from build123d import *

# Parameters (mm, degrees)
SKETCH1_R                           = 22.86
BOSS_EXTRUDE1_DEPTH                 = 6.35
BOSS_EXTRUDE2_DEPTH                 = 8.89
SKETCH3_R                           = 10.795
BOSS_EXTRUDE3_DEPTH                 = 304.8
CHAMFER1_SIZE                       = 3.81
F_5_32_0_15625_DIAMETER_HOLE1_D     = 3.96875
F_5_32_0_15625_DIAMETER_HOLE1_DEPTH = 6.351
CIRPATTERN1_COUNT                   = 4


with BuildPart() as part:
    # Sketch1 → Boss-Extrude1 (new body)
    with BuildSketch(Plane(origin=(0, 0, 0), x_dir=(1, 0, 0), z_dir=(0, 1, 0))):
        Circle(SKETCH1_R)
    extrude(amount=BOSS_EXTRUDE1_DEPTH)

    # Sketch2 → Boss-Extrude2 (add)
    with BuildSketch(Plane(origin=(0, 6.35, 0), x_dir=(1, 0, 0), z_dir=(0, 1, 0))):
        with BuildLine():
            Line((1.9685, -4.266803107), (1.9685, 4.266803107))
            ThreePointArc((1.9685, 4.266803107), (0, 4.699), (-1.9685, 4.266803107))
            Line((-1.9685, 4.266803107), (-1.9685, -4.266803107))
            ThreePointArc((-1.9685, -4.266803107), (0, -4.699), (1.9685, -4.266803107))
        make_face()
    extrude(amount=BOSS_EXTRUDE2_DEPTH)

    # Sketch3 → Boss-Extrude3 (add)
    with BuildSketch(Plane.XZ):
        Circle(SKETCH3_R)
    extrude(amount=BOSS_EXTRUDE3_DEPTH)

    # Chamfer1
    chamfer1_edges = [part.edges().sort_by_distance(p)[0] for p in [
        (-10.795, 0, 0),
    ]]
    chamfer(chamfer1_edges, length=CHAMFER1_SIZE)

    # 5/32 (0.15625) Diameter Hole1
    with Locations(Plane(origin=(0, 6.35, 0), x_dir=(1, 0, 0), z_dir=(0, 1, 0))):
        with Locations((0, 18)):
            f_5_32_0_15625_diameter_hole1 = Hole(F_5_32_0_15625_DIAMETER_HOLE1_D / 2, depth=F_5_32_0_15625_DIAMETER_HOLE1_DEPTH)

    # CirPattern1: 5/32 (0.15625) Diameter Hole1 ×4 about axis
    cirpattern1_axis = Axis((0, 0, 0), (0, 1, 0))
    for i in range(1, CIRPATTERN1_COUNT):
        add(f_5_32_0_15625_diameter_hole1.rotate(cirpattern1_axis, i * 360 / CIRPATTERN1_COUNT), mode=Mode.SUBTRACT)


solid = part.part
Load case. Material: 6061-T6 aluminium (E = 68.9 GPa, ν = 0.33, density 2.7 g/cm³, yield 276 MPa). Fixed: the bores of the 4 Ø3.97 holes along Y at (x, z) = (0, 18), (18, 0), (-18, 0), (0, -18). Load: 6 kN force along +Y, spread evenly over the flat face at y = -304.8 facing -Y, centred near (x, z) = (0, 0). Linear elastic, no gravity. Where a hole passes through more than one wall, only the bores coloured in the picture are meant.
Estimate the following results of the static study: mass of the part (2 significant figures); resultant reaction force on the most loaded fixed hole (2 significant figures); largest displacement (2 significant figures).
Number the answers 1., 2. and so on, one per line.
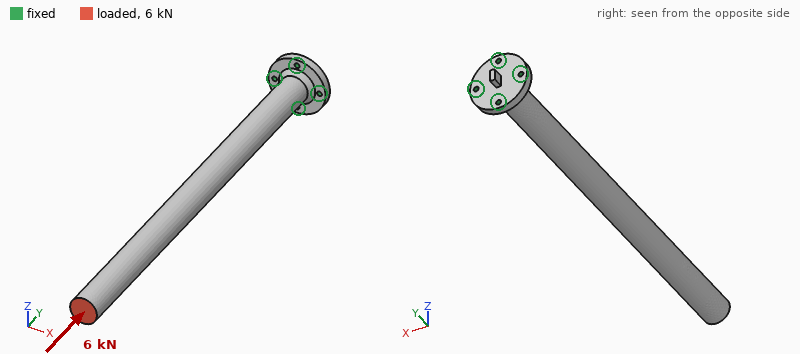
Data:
1. 330 g
2. 1.6 kN
3. 80 µm
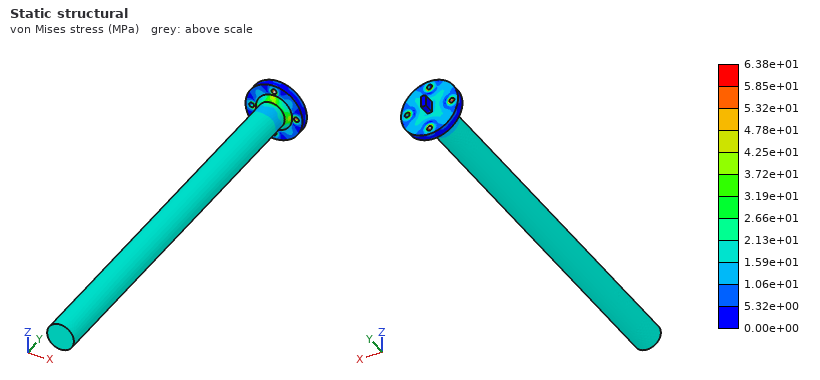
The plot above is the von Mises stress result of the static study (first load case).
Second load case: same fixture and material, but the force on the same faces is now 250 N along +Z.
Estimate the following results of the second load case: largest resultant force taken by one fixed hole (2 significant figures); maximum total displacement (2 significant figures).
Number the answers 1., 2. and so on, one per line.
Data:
1. 2.2 kN
2. 3.4 mm
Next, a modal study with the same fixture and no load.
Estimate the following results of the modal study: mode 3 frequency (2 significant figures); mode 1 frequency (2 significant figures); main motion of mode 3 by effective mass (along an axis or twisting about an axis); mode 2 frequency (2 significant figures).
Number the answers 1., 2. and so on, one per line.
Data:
1. 980 Hz
2. 160 Hz
3. along Z
4. 160 Hz
